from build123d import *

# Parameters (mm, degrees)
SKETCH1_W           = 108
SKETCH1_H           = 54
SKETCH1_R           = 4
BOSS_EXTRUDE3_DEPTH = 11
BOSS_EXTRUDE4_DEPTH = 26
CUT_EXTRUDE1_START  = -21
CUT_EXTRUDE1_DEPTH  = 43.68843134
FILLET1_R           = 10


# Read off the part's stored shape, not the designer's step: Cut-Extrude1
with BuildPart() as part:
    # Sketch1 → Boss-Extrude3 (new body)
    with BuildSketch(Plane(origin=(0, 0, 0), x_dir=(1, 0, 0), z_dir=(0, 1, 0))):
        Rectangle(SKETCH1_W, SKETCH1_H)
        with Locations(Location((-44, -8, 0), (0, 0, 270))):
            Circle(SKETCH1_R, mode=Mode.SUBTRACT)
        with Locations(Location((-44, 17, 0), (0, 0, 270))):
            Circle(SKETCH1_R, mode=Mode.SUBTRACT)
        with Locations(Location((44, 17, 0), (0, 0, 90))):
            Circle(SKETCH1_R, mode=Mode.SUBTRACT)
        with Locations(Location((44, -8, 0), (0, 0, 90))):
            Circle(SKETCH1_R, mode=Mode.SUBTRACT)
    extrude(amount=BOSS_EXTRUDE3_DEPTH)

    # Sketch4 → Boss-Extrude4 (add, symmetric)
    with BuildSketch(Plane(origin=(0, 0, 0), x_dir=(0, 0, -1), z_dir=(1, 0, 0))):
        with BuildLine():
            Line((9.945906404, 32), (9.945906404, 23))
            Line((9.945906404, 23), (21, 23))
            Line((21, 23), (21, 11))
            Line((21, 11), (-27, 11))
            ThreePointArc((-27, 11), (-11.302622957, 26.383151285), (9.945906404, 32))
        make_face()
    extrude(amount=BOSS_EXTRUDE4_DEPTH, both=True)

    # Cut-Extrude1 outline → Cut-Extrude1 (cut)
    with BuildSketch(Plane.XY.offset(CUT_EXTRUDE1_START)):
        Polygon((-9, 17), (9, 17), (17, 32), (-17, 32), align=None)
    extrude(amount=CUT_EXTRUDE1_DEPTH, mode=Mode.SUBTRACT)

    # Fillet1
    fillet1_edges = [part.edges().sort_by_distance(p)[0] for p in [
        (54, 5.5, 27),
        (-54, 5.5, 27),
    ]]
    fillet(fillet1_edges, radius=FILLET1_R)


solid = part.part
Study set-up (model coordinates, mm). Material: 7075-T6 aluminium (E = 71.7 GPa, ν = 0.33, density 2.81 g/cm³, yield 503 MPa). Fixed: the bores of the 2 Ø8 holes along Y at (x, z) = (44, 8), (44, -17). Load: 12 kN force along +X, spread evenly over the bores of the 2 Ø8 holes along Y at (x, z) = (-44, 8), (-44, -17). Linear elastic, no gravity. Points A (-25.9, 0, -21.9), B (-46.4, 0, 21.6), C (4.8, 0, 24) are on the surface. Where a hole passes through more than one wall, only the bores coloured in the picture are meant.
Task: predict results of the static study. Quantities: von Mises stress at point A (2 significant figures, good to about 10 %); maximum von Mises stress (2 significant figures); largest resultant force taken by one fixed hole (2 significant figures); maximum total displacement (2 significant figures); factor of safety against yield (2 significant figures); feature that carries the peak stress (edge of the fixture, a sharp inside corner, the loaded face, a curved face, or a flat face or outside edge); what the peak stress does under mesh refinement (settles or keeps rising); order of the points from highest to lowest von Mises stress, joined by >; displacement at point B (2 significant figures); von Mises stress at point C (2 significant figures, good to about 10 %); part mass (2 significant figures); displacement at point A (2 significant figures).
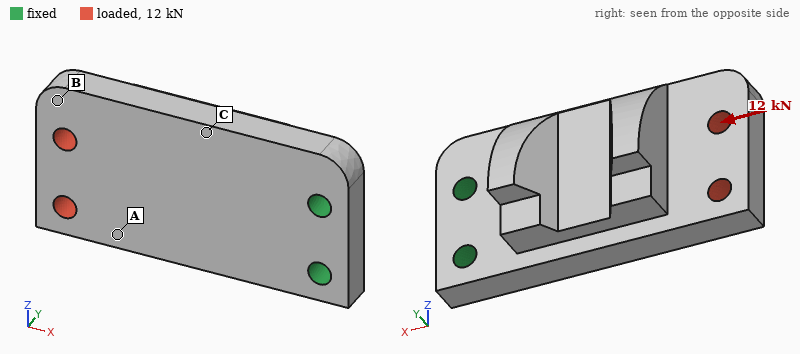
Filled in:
29 MPa
66 MPa
6.1 kN
69 µm
7.6
the loaded face
settles
A > C > B
51 µm
18 MPa
250 g
41 µm
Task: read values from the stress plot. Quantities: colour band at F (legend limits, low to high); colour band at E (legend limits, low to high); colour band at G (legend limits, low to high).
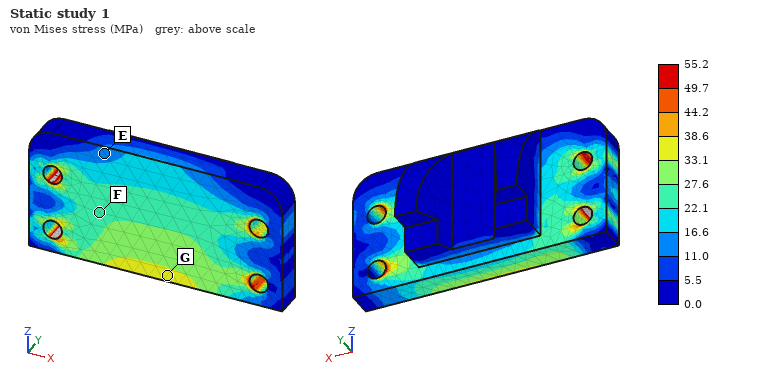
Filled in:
22.1 to 27.6 MPa
11.0 to 16.6 MPa
33.1 to 38.6 MPa
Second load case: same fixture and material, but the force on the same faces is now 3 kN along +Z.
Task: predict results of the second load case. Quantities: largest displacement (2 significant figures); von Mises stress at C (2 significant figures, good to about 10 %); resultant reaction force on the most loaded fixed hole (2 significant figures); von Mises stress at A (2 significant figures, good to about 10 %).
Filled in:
0.12 mm
20 MPa
8.6 kN
10 MPa
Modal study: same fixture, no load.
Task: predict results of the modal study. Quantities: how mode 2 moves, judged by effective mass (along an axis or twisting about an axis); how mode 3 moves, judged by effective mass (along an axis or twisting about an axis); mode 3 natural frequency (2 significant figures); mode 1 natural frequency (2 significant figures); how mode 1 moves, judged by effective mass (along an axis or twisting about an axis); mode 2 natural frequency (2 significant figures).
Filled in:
along Z
twisting about X
4200 Hz
990 Hz
along Y
3100 Hz
